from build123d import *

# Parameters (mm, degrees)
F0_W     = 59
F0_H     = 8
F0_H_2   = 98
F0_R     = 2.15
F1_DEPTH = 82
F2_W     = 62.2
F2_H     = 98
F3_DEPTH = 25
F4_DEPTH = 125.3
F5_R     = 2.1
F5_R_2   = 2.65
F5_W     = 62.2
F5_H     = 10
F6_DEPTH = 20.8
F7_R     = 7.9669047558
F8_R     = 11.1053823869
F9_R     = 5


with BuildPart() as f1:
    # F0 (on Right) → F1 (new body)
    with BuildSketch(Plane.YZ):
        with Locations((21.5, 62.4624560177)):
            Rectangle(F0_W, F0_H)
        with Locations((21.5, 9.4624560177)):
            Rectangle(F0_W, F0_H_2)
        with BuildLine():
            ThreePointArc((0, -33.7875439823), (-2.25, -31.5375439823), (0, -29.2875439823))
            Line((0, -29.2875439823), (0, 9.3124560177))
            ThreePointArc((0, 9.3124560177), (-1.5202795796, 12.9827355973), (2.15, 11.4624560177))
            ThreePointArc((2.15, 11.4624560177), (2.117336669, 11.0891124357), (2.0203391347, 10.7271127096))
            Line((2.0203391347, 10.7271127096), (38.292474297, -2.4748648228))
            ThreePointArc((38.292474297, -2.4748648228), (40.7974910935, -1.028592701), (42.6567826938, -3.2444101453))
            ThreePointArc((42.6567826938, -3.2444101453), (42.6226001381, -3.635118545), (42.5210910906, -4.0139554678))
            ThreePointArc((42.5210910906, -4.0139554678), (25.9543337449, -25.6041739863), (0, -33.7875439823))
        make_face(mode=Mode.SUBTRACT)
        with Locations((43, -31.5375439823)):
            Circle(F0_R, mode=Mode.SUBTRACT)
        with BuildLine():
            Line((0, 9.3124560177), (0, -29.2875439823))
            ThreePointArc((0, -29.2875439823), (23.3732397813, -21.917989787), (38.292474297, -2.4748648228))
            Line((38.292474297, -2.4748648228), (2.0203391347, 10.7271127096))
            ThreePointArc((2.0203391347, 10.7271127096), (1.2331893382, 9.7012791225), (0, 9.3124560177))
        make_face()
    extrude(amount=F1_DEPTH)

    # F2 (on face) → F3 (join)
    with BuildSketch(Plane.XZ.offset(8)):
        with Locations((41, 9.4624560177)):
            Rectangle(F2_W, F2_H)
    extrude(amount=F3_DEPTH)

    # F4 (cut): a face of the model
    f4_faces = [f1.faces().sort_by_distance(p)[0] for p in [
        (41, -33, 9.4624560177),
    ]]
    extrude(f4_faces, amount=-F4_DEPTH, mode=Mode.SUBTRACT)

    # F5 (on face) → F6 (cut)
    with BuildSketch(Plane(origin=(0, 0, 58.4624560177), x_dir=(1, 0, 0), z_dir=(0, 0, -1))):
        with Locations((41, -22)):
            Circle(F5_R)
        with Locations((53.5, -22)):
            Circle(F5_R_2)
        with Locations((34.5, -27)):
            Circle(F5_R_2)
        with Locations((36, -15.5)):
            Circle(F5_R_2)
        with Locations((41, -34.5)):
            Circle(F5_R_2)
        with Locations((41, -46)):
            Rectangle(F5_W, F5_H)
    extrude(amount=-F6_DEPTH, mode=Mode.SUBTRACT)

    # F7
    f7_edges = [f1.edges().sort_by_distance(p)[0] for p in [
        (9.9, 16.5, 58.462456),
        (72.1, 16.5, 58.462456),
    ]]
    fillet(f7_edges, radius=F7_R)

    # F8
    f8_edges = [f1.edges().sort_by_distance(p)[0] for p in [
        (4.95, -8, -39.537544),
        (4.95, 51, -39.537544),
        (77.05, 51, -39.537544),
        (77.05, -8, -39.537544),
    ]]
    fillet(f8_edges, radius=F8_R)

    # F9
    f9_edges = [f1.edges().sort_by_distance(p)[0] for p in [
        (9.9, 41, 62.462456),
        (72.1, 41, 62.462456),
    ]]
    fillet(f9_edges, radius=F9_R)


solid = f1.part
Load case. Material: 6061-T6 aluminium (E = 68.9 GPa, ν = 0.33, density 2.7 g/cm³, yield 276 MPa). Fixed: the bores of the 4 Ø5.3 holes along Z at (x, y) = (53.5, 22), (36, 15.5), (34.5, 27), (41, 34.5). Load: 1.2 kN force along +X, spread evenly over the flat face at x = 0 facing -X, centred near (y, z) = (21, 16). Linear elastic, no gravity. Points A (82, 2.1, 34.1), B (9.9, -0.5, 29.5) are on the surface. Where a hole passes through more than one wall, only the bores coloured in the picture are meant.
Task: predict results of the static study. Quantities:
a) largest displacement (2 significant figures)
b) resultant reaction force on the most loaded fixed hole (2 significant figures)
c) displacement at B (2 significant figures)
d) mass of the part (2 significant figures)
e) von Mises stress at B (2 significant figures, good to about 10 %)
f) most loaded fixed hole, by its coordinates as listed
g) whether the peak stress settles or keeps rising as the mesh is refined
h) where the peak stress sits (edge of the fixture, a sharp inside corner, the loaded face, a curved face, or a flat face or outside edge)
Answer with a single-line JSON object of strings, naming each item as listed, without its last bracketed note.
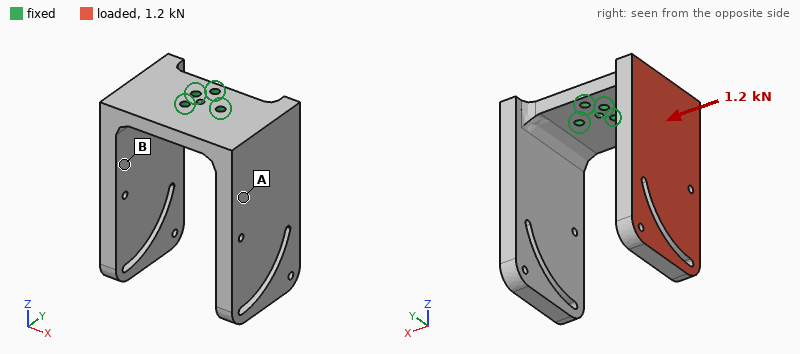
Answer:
{"largest displacement": "1.3 mm", "resultant reaction force on the most loaded fixed hole": "1.1 kN", "displacement at B": "0.36 mm", "mass of the part": "380 g", "von Mises stress at B": "26 MPa", "most loaded fixed hole, by its coordinates as listed": "(34.5, 27)", "whether the peak stress settles or keeps rising as the mesh is refined": "keeps rising", "where the peak stress sits": "edge of the fixture"}
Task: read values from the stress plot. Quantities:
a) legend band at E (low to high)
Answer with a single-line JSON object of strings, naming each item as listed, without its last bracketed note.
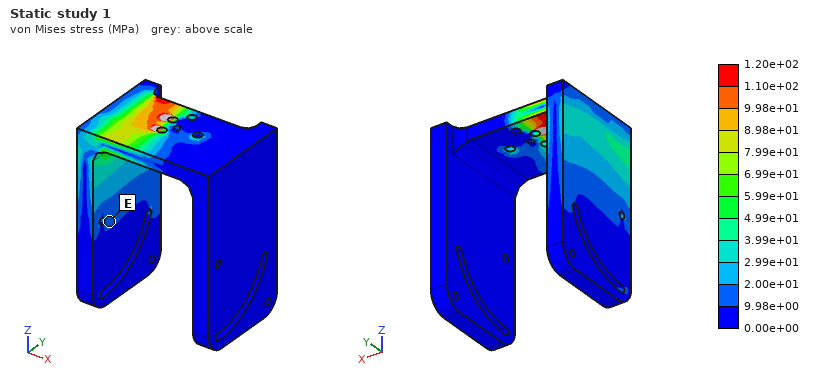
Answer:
{"legend band at E": "9.98e+00 to 2.00e+01 MPa"}
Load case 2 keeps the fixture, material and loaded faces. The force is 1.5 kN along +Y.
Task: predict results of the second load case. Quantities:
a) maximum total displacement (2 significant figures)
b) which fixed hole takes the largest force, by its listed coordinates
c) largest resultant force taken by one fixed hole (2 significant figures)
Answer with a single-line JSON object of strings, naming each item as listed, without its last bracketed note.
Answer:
{"maximum total displacement": "0.57 mm", "which fixed hole takes the largest force, by its listed coordinates": "(36, 15.5)", "largest resultant force taken by one fixed hole": "3.5 kN"}
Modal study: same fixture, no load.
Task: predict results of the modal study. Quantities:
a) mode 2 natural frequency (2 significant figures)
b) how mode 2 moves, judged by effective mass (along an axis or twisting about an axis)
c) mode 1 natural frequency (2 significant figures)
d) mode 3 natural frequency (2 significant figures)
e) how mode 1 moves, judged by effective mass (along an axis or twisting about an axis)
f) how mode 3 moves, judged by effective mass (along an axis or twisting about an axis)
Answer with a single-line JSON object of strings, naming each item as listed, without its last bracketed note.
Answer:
{"mode 2 natural frequency": "510 Hz", "how mode 2 moves, judged by effective mass": "along X", "mode 1 natural frequency": "470 Hz", "mode 3 natural frequency": "760 Hz", "how mode 1 moves, judged by effective mass": "along X", "how mode 3 moves, judged by effective mass": "along Y"}
